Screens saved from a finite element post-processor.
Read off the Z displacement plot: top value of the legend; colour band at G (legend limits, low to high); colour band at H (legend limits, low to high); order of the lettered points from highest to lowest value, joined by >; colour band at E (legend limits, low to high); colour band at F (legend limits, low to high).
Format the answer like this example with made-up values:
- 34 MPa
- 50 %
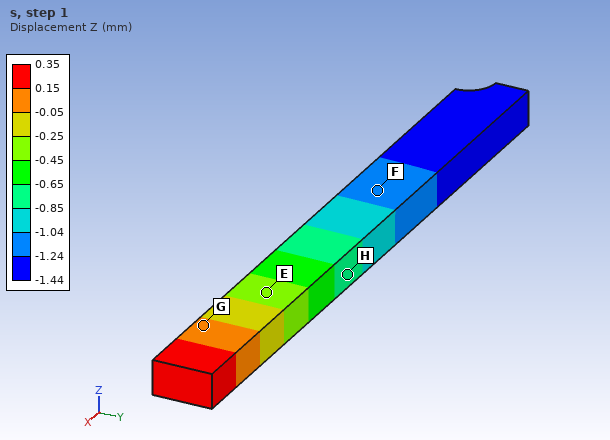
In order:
- 0.35 mm
- -0.05 to 0.15 mm
- -0.85 to -0.65 mm
- G > E > H > F
- -0.45 to -0.25 mm
- -1.24 to -1.04 mm
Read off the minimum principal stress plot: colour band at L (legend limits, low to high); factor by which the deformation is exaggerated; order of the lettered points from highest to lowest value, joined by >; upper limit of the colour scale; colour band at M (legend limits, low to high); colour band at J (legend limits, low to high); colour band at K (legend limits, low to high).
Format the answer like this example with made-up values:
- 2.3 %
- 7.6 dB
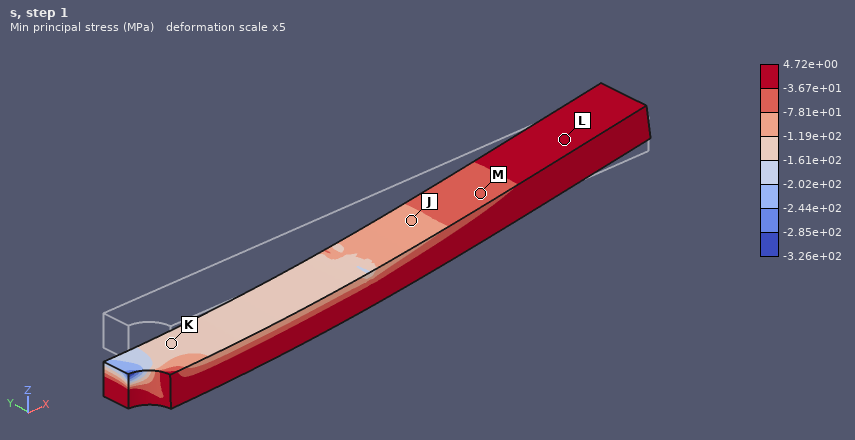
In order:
- -3.67e+01 to 4.72e+00 MPa
- 5
- L > M > J > K
- 4.72e+00 MPa
- -7.81e+01 to -3.67e+01 MPa
- -1.19e+02 to -7.81e+01 MPa
- -1.61e+02 to -1.19e+02 MPa
